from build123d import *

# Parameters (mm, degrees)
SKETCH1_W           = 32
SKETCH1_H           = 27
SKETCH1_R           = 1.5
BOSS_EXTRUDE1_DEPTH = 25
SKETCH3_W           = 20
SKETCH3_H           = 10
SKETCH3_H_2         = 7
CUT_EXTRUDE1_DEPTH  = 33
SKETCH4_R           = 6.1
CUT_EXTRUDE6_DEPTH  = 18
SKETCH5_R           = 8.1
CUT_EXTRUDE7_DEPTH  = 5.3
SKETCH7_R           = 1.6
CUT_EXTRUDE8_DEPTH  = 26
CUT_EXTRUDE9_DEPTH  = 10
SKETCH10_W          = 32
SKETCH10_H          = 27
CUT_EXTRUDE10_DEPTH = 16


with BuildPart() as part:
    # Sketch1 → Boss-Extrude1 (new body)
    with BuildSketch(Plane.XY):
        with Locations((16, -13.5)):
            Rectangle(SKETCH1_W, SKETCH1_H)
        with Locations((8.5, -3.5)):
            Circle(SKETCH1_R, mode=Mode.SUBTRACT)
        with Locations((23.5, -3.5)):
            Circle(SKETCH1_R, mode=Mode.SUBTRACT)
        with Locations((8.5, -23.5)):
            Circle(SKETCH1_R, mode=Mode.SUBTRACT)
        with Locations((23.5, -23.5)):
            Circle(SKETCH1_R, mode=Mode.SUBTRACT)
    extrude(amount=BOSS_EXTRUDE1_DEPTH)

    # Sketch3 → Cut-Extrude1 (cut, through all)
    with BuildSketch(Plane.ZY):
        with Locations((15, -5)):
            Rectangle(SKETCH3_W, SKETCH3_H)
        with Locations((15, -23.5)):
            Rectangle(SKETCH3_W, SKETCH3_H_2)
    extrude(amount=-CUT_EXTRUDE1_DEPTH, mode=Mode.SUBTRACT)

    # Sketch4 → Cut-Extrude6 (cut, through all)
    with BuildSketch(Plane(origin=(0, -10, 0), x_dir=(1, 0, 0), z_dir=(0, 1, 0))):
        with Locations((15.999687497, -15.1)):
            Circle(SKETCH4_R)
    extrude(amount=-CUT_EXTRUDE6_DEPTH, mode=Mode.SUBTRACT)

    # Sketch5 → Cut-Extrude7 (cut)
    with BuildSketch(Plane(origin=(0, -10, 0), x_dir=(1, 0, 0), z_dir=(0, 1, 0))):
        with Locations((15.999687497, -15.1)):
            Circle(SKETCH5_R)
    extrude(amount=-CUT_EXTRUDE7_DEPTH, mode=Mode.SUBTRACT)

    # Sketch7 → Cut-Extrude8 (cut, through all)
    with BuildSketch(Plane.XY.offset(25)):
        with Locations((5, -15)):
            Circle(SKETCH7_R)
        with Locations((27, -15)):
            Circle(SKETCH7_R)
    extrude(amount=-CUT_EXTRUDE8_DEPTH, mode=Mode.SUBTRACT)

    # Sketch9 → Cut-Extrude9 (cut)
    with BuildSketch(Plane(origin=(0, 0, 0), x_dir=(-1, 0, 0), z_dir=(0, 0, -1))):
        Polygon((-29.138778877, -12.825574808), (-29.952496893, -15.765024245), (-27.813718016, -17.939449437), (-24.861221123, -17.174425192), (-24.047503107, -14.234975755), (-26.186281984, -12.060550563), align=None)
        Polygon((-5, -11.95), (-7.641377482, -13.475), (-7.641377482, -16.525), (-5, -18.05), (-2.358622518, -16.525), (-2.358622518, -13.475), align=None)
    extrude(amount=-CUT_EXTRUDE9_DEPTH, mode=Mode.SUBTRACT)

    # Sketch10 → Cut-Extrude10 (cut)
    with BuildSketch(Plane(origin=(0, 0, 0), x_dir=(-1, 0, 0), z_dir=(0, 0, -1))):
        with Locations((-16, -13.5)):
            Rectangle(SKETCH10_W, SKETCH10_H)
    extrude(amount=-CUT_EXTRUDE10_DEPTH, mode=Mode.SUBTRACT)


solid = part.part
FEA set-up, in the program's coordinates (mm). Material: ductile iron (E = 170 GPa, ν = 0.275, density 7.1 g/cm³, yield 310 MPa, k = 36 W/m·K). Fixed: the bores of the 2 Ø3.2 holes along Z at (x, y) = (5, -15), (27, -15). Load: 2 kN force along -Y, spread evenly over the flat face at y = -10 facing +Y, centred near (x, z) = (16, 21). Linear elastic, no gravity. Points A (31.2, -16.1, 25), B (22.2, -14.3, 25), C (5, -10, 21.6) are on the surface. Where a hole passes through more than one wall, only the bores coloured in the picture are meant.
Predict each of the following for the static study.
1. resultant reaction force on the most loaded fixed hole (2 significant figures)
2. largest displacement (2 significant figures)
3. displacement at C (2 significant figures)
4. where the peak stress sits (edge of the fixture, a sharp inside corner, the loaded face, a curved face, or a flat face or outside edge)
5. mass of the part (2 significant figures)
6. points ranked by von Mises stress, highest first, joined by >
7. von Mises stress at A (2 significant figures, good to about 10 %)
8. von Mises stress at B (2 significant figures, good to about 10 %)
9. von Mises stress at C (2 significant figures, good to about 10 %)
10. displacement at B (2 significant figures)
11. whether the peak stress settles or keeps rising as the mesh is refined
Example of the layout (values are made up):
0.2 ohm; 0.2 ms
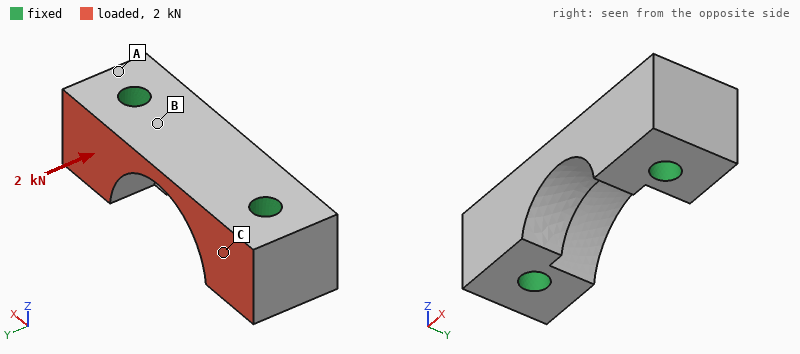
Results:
1.0 kN; 1.4 µm; 0.30 µm; edge of the fixture; 15 g; C > B > A; 4.6 MPa; 12 MPa; 18 MPa; 0.64 µm; keeps rising
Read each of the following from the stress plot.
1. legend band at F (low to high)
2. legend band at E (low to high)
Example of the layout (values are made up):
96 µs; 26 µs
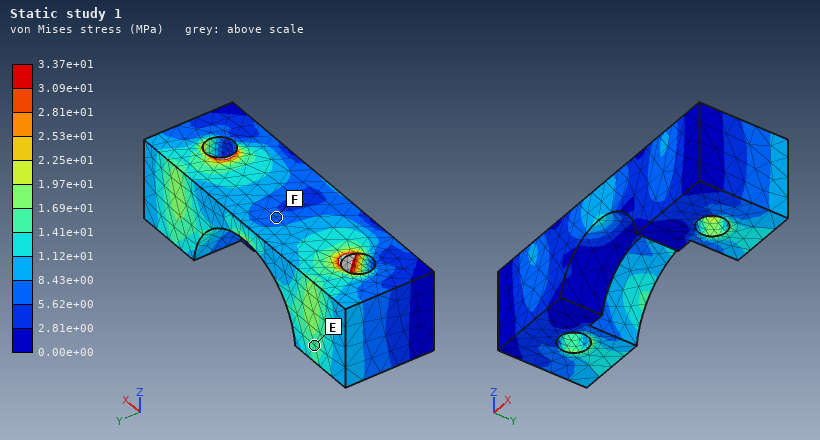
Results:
5.62e+00 to 8.43e+00 MPa; 1.41e+01 to 1.69e+01 MPa
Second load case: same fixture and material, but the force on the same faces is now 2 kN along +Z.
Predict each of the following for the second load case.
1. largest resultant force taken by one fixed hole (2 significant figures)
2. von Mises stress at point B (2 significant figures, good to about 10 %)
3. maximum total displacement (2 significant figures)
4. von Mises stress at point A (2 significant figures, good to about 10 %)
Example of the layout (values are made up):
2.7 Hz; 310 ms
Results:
1.0 kN; 24 MPa; 4.9 µm; 9.8 MPa
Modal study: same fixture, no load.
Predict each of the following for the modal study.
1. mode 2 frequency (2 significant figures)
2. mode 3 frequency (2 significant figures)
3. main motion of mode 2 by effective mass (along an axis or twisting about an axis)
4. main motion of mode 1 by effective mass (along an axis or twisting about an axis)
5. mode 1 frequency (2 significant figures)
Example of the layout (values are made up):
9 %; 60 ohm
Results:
65 kHz; 83 kHz; along Z; along Y; 55 kHz
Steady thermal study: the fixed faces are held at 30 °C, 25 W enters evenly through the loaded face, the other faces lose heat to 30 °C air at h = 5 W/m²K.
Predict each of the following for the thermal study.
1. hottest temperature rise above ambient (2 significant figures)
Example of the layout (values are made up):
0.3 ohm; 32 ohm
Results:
25 K
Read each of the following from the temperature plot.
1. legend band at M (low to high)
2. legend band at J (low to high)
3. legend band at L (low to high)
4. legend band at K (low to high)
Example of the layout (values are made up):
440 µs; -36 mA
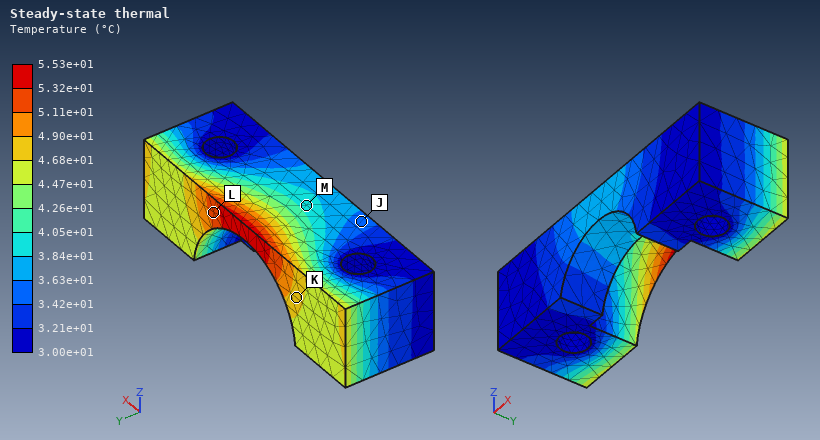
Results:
3.84e+01 to 4.05e+01 °C; 3.42e+01 to 3.63e+01 °C; 5.11e+01 to 5.32e+01 °C; 4.68e+01 to 4.90e+01 °C
